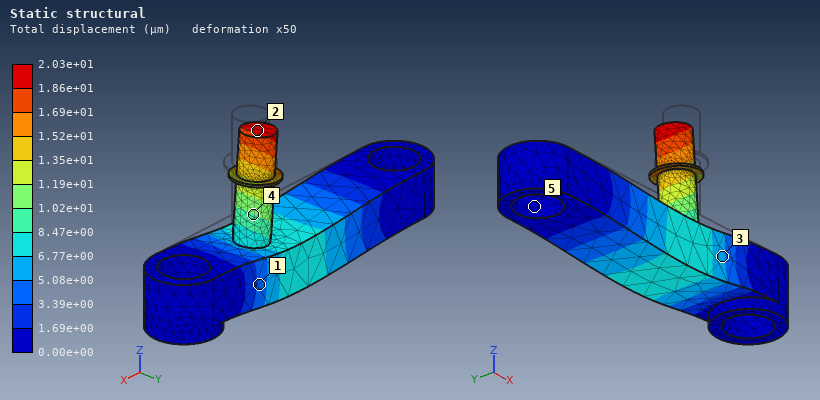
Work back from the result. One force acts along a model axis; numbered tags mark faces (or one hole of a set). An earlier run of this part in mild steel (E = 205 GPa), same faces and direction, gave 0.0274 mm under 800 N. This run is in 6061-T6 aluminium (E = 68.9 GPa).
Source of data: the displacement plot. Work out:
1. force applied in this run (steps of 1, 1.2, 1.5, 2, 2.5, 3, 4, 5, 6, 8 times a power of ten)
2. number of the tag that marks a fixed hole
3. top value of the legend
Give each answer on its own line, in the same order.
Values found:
200 N
5
2.03e+01 µm
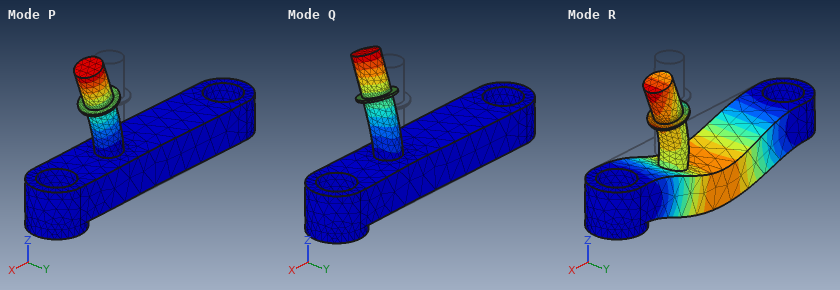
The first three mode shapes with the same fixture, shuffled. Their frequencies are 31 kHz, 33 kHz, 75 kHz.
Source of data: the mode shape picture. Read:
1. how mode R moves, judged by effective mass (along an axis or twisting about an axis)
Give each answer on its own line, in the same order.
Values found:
along Z
